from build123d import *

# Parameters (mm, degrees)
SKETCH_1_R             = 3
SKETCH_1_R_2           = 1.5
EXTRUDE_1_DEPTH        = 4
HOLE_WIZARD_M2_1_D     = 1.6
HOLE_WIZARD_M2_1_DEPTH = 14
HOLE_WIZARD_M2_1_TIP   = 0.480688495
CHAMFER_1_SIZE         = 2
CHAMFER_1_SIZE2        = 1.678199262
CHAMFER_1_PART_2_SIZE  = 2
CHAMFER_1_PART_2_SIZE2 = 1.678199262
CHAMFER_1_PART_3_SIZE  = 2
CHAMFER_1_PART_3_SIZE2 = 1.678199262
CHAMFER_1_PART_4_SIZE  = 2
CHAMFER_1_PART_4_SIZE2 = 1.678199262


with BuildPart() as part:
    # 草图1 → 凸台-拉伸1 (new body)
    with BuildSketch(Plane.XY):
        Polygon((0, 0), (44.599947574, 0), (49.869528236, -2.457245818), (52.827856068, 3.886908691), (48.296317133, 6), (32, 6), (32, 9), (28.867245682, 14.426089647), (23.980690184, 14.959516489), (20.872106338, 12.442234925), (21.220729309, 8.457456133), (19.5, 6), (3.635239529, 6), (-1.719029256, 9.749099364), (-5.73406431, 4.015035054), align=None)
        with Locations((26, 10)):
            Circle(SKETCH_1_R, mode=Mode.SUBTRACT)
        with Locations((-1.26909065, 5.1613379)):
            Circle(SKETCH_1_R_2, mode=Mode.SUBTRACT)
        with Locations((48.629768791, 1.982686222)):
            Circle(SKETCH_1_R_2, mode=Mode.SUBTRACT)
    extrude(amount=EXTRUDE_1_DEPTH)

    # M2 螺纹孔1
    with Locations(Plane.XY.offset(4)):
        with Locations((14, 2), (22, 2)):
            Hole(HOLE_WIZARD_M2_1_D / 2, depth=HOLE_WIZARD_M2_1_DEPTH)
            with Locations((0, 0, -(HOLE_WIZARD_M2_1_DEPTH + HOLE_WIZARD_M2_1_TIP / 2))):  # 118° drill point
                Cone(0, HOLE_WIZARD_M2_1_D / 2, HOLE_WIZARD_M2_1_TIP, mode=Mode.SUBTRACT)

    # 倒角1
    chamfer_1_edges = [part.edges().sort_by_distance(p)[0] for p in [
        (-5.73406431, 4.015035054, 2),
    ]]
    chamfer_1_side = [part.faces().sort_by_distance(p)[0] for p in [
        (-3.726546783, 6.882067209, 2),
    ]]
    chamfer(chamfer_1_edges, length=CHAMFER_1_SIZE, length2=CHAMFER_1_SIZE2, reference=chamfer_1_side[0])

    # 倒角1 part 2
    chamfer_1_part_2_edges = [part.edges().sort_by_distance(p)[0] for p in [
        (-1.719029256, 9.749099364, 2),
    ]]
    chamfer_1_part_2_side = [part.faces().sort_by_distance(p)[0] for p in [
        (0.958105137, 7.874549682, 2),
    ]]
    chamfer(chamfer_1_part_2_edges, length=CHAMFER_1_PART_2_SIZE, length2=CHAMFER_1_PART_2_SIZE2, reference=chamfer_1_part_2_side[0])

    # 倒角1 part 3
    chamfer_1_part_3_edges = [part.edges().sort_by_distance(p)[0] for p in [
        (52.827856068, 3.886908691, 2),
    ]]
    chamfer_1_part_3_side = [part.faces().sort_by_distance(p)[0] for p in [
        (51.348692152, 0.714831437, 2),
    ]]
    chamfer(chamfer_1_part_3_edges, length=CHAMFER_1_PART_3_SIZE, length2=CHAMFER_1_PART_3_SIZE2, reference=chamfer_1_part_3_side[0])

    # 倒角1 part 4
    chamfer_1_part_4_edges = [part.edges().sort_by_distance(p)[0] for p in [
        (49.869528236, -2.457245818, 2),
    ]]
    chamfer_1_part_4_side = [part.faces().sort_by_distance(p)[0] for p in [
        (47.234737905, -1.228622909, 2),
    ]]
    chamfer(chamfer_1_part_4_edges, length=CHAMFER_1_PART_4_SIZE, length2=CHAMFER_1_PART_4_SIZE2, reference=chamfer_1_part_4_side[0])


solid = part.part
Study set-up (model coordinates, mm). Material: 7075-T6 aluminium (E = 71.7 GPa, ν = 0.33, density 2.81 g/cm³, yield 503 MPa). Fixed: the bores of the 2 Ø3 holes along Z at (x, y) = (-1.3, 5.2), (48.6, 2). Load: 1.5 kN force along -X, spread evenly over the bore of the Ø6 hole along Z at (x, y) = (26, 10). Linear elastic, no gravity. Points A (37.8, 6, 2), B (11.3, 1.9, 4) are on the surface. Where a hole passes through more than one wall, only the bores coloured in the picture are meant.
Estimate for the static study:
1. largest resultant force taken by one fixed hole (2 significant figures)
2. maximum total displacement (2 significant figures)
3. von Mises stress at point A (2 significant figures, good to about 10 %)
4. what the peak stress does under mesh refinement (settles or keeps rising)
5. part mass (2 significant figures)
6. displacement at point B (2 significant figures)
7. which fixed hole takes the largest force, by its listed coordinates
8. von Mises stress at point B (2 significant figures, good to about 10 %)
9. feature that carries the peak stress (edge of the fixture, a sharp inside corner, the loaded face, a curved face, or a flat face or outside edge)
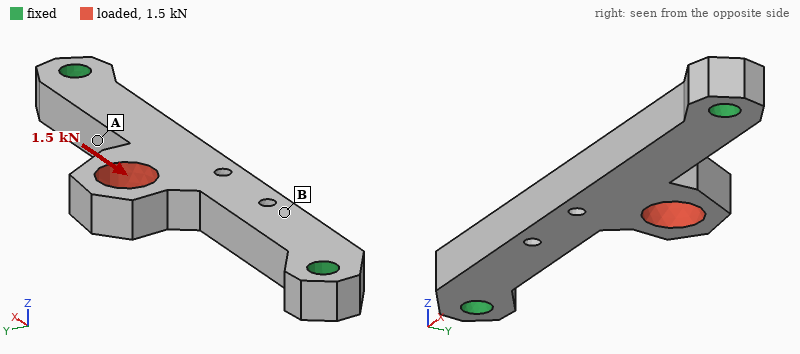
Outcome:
990 N
89 µm
96 MPa
keeps rising
4.3 g
35 µm
(48.6, 2)
35 MPa
a sharp inside corner
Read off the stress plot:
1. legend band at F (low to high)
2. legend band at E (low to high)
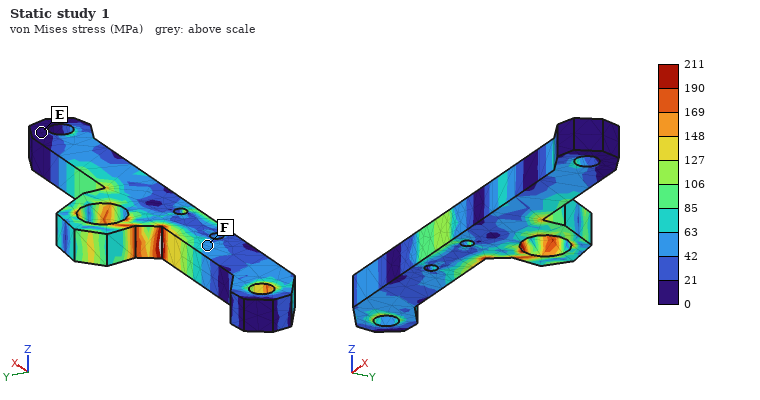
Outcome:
42 to 63 MPa
0 to 21 MPa
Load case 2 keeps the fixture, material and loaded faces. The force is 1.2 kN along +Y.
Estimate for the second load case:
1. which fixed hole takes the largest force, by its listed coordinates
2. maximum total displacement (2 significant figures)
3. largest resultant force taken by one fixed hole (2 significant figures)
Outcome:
(48.6, 2)
0.14 mm
680 N
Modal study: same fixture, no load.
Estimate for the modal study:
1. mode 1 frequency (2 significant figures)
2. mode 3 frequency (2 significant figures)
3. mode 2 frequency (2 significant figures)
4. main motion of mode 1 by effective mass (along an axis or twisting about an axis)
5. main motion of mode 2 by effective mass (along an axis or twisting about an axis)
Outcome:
6800 Hz
13 kHz
10 kHz
along Z
along Y
